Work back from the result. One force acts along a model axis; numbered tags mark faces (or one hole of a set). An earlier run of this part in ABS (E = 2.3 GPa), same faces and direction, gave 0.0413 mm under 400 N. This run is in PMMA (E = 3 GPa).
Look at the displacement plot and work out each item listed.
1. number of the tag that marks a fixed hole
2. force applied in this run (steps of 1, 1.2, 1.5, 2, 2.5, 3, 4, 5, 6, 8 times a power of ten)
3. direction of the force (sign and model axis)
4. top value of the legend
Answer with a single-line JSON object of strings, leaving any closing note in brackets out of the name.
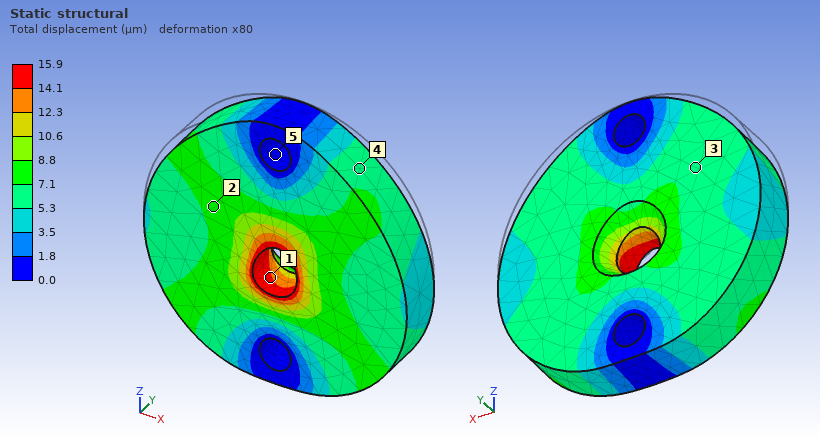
{"number of the tag that marks a fixed hole": "5", "force applied in this run": "200 N", "direction of the force": "-Z", "top value of the legend": "15.9 µm"}
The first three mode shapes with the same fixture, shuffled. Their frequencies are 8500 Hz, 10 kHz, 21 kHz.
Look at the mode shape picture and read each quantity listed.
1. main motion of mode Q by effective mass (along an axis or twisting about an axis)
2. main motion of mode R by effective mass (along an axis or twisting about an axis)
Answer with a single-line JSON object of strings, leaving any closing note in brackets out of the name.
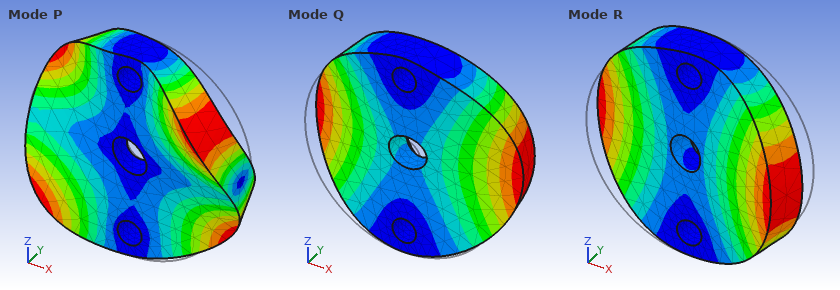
{"main motion of mode Q by effective mass": "along Y", "main motion of mode R by effective mass": "twisting about Z"}
